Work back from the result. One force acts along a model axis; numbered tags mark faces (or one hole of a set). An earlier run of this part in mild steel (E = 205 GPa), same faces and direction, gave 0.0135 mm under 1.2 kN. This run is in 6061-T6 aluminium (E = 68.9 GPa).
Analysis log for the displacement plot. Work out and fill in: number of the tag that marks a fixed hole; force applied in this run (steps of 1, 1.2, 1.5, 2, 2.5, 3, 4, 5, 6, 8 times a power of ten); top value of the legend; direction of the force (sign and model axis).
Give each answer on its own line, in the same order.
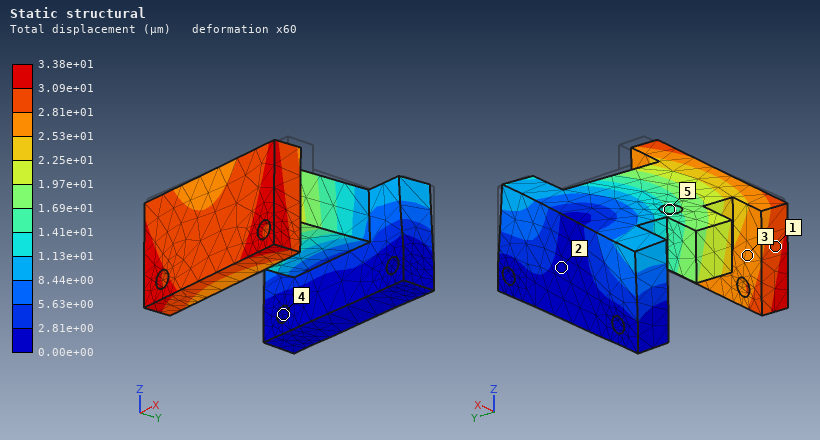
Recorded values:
4
1 kN
3.38e+01 µm
-X
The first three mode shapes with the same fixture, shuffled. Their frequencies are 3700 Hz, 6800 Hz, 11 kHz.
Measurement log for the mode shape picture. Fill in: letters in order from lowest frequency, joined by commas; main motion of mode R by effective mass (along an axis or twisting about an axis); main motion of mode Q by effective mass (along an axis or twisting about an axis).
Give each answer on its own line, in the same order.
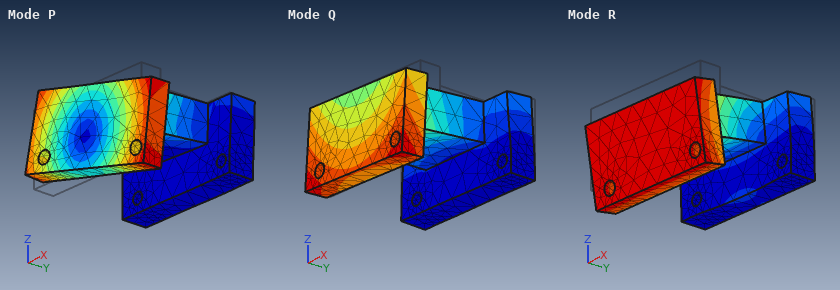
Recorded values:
R, Q, P
along Z
along X
